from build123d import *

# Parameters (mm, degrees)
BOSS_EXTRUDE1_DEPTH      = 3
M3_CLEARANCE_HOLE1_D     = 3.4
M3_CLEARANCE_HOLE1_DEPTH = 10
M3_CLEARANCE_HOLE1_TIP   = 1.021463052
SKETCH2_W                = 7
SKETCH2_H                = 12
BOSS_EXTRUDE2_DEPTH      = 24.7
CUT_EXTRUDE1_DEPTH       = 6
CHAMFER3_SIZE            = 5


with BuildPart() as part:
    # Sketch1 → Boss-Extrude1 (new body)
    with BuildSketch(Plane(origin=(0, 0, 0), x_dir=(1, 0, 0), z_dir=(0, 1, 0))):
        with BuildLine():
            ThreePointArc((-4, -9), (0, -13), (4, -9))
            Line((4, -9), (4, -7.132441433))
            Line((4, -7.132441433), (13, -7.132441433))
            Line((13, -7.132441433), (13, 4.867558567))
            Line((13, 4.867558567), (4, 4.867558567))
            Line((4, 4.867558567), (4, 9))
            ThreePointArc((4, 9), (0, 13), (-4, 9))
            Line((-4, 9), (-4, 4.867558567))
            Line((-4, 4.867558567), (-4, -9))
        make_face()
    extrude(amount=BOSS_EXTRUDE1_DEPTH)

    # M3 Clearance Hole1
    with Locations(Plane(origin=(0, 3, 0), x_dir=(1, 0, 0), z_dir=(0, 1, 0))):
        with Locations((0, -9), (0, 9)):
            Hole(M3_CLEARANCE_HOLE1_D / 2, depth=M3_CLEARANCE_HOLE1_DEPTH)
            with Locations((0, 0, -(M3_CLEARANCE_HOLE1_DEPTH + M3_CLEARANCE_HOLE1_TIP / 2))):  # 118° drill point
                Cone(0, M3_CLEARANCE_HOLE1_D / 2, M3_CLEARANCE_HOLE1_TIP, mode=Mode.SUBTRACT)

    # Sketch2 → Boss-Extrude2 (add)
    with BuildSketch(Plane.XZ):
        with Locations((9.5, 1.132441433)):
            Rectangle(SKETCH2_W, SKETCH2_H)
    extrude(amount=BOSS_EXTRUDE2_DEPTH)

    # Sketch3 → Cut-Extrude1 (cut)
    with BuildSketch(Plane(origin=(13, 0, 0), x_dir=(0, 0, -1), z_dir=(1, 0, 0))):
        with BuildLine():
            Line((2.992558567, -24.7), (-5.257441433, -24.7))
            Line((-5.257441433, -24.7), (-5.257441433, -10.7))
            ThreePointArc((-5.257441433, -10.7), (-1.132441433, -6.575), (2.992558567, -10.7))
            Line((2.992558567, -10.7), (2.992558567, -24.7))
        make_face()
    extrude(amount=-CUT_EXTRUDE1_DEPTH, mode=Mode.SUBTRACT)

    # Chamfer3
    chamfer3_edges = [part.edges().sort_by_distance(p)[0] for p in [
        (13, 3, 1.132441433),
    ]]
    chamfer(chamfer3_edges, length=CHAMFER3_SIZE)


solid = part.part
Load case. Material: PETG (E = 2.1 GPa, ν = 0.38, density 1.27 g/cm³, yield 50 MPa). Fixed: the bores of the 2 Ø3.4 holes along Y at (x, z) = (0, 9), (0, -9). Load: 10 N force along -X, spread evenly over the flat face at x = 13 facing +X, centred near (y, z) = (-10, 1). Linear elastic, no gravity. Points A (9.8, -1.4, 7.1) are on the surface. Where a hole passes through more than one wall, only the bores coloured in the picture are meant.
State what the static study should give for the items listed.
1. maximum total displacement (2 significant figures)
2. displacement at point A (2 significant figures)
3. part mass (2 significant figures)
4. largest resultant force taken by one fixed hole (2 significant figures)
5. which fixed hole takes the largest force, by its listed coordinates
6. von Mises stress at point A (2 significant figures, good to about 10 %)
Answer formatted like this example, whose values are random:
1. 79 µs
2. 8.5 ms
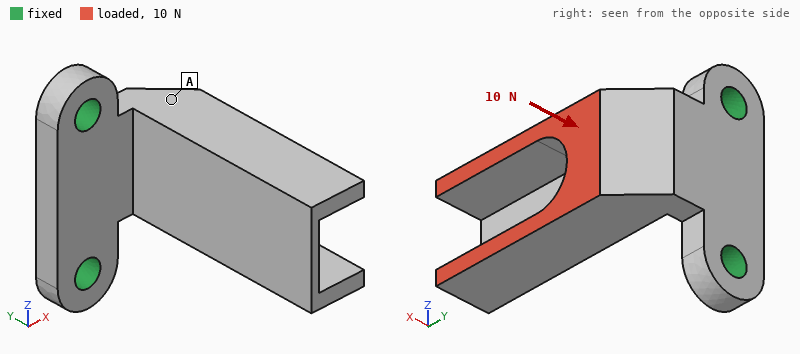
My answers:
1. 0.49 mm
2. 0.11 mm
3. 2.4 g
4. 6.1 N
5. (0, 9)
6. 1.3 MPa
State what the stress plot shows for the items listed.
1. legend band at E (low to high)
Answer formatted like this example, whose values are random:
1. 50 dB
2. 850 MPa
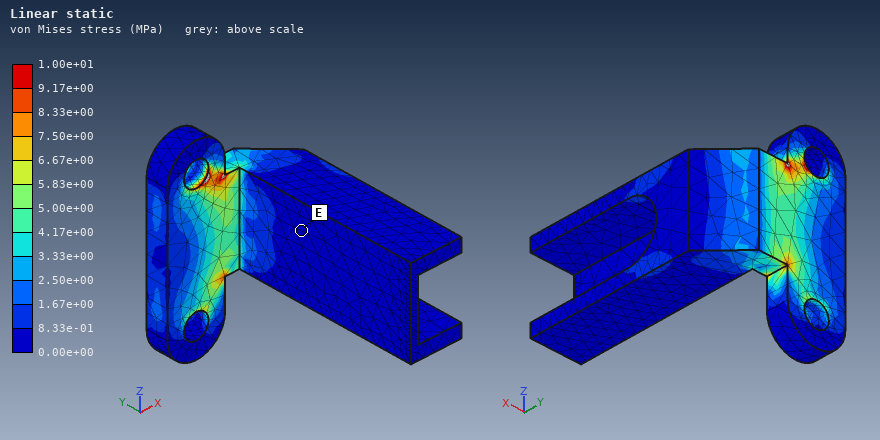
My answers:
1. 0.00e+00 to 8.33e-01 MPa
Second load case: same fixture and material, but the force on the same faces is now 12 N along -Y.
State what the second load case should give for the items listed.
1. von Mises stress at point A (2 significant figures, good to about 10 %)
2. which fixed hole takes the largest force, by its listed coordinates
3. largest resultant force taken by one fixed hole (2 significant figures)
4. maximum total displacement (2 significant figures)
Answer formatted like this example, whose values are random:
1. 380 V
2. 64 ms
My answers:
1. 1.00 MPa
2. (0, 9)
3. 7.1 N
4. 0.46 mm
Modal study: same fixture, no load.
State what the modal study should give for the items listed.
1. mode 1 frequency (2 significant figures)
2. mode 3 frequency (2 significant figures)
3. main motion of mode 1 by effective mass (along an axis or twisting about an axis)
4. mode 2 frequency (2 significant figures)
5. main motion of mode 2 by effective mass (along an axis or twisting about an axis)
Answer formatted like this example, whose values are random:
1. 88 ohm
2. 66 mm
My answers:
1. 720 Hz
2. 3200 Hz
3. along X
4. 1300 Hz
5. along Z
